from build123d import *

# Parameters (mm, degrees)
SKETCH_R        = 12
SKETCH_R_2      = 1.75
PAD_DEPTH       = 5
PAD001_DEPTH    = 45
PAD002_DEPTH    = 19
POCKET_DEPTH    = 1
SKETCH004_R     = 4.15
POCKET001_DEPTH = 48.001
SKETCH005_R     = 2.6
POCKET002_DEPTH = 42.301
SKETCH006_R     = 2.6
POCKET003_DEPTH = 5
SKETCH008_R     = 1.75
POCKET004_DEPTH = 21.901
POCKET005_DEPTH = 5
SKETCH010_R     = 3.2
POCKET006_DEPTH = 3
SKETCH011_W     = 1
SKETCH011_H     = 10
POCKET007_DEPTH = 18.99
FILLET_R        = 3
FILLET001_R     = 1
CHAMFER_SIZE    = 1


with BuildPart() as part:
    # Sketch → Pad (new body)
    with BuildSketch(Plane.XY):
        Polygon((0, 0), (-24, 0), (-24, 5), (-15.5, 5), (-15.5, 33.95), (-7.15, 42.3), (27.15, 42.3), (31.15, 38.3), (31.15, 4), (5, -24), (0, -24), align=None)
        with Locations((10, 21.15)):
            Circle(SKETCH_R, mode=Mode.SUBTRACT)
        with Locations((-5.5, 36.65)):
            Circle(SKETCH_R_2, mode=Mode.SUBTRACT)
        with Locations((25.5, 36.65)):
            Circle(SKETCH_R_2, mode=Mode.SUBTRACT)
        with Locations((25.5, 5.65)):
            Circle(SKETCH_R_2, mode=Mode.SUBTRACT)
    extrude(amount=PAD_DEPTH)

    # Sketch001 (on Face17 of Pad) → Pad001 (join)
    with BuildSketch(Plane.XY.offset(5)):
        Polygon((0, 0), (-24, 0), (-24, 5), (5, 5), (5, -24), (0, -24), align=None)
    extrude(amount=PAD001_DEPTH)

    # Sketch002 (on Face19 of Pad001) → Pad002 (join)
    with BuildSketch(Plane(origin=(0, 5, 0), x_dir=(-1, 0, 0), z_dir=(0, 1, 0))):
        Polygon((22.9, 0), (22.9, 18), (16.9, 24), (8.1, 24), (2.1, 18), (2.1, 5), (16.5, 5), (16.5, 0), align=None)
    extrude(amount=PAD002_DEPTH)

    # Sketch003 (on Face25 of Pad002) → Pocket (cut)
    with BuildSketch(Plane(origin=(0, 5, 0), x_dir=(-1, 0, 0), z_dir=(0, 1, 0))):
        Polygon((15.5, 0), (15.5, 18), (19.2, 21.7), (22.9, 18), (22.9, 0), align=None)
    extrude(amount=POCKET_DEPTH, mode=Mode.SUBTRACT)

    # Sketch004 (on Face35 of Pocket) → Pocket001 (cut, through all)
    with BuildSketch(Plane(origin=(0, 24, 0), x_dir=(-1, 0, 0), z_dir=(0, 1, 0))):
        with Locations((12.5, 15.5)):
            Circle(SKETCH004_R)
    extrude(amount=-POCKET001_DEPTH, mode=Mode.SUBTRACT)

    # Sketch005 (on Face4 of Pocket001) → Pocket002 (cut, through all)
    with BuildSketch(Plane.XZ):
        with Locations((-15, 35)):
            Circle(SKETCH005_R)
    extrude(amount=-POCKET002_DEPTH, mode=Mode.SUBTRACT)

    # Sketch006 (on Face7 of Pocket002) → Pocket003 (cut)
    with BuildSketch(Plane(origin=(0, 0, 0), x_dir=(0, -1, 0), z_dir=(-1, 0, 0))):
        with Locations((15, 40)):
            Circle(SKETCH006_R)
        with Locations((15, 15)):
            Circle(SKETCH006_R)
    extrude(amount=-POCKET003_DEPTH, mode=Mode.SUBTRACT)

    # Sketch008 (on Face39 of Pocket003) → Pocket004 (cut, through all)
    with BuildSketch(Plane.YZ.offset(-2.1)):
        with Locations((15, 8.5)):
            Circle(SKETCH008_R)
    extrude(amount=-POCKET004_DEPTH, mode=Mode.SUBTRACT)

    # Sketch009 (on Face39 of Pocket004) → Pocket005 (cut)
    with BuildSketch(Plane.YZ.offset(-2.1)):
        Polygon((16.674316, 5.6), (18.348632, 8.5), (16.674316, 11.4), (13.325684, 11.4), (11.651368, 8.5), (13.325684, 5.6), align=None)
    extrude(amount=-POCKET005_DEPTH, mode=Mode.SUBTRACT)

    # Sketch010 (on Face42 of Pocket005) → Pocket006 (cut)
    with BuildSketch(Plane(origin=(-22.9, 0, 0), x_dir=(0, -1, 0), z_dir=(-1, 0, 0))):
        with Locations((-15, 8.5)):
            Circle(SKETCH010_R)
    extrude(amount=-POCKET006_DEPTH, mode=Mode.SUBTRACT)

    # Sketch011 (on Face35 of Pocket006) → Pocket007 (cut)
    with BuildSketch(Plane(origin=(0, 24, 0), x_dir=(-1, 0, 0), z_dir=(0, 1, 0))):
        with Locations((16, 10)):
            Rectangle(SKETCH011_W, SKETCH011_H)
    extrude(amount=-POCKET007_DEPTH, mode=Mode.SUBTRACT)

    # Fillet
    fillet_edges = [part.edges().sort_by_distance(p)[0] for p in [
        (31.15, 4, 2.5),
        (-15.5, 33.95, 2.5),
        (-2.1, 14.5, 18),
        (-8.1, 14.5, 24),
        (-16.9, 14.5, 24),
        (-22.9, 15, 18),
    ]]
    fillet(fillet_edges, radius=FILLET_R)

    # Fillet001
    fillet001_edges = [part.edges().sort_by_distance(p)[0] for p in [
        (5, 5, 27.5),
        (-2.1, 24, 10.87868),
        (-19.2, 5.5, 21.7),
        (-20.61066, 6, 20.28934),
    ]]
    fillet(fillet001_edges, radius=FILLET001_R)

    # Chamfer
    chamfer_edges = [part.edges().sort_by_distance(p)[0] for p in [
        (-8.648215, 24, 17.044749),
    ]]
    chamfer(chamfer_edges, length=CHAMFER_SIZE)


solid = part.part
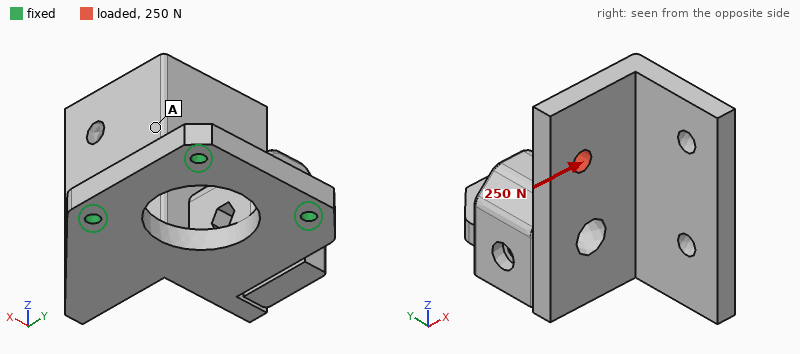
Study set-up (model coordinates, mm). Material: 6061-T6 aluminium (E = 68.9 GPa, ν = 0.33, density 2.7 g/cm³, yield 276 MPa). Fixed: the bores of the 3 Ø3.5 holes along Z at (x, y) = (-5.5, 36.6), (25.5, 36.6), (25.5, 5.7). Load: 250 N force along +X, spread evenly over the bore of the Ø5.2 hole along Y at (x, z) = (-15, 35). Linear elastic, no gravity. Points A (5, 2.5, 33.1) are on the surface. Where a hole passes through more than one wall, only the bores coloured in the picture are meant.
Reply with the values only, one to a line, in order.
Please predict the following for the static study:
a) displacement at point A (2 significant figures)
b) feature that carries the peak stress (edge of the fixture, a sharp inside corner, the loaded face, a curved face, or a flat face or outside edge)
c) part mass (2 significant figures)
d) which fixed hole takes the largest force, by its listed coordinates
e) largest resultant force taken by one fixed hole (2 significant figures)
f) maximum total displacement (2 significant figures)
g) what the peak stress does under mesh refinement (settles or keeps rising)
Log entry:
0.14 mm
edge of the fixture
71 g
(25.5, 5.7)
230 N
0.26 mm
keeps rising
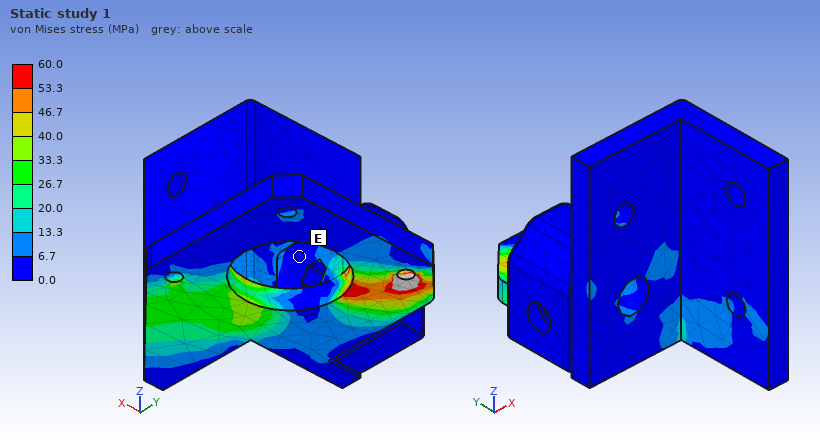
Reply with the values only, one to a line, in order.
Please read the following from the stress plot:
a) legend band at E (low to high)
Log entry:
0.0 to 6.7 MPa
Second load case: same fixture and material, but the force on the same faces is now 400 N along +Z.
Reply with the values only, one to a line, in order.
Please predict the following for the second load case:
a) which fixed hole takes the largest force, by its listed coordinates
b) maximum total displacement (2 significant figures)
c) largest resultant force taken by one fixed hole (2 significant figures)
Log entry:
(-5.5, 36.6)
0.38 mm
280 N
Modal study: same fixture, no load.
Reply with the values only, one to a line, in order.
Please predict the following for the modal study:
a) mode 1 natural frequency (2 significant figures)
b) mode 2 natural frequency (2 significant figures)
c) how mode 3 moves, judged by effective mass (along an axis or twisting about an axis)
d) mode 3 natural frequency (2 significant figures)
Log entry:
880 Hz
2200 Hz
along Z
4000 Hz
